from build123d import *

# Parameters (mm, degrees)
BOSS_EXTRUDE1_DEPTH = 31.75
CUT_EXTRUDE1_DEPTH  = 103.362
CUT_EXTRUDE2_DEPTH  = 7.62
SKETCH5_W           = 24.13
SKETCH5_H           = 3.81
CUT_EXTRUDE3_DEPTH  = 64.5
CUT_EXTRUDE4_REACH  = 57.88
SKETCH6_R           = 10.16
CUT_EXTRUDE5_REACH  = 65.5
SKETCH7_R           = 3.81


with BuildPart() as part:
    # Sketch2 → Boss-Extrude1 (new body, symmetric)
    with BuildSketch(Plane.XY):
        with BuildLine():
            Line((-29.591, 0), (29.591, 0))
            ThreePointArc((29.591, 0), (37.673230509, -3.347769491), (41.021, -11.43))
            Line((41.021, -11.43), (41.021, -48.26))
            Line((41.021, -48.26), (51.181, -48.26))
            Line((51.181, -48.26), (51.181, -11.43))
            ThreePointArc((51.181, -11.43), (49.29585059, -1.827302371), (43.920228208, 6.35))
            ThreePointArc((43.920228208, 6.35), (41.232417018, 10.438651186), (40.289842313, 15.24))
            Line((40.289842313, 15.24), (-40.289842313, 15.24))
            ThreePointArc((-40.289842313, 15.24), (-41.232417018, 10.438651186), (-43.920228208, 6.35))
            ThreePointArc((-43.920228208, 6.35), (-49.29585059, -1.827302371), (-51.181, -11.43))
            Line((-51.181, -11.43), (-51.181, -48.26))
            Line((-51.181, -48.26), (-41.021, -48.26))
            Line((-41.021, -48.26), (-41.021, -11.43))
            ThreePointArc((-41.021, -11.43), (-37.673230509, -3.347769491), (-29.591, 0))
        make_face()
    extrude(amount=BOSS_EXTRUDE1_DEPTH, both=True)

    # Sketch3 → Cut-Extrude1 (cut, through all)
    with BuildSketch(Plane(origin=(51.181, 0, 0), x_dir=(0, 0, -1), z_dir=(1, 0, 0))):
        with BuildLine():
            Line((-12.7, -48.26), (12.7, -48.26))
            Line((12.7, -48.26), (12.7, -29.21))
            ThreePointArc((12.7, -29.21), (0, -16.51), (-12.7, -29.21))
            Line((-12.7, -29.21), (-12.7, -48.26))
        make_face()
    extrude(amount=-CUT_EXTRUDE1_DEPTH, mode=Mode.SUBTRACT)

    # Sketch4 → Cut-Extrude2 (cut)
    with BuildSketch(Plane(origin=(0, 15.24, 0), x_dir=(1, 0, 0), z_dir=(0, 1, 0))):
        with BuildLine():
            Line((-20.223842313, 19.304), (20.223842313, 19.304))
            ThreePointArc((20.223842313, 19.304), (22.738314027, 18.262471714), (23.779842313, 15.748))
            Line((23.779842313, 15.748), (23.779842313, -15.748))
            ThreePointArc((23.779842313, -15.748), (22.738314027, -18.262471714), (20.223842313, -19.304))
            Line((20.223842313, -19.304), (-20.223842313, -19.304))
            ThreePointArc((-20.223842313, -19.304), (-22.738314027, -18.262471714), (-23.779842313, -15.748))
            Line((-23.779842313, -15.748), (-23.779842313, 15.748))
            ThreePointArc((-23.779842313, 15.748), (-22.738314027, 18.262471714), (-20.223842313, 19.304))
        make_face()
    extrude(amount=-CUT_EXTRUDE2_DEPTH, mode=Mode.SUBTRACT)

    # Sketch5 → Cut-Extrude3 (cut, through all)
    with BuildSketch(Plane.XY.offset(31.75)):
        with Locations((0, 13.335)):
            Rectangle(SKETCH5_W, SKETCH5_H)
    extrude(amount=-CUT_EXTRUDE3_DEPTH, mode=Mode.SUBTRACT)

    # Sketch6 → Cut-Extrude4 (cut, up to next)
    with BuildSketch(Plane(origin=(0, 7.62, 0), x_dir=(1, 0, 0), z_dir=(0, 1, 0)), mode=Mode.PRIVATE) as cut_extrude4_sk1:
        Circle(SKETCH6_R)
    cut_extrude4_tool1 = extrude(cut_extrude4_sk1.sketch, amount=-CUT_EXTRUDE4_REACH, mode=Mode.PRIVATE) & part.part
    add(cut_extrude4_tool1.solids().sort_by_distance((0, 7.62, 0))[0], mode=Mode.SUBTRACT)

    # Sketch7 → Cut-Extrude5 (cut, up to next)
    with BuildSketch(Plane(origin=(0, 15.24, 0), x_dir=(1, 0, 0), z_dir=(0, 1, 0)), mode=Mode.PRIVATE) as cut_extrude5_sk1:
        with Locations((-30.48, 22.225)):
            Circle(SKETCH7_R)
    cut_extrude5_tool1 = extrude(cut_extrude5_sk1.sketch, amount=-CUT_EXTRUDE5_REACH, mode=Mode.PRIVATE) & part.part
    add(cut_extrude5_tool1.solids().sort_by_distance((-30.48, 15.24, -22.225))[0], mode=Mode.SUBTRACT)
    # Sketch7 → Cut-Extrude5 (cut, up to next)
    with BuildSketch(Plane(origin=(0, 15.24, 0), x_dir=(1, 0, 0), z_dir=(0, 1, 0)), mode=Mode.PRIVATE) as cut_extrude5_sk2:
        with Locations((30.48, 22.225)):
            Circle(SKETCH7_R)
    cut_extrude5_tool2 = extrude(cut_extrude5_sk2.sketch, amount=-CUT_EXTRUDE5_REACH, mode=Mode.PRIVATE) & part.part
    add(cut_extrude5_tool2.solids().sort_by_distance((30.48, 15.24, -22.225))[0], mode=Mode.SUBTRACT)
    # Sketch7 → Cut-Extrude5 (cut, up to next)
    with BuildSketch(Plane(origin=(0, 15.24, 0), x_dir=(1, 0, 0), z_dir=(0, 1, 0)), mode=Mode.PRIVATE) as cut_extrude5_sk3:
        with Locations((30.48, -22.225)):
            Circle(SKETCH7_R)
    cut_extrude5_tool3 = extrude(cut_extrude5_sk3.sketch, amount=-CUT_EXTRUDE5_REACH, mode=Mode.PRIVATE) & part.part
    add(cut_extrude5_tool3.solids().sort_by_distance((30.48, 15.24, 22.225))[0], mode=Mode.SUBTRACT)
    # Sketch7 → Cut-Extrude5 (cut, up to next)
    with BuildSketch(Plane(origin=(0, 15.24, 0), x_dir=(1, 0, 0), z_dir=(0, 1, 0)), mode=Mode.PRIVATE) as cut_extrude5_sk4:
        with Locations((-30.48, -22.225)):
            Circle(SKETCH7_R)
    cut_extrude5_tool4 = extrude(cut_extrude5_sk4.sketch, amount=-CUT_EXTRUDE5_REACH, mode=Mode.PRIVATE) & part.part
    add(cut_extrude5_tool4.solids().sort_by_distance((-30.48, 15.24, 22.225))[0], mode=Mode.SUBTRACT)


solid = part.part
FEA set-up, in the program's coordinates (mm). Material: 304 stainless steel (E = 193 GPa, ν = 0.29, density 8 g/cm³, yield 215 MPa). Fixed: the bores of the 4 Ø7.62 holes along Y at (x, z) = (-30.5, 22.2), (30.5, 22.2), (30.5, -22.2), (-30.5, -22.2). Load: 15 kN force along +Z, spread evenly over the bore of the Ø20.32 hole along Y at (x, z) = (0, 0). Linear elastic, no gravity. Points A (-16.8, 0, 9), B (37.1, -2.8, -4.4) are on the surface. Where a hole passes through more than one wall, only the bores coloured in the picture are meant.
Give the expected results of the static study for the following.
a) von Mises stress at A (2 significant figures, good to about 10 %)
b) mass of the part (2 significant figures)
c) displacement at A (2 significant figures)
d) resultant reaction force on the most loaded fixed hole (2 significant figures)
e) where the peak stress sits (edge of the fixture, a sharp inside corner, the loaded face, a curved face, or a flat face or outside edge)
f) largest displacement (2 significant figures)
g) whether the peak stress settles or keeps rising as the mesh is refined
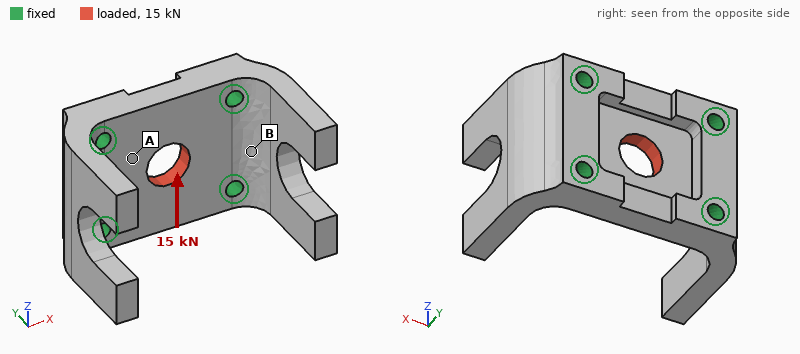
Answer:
27 MPa
900 g
2.7 µm
4.3 kN
edge of the fixture
6.5 µm
keeps rising
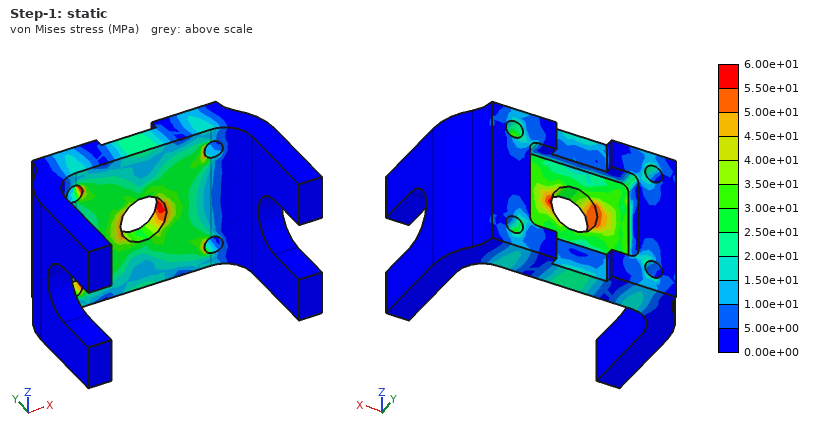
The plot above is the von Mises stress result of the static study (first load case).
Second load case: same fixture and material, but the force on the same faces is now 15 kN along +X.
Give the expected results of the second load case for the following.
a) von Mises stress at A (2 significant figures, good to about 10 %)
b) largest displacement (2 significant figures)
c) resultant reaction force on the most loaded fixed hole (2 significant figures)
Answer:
23 MPa
3.8 µm
3.9 kN
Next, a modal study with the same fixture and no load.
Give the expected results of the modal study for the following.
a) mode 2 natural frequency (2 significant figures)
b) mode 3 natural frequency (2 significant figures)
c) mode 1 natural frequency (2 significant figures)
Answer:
3100 Hz
3700 Hz
3100 Hz
